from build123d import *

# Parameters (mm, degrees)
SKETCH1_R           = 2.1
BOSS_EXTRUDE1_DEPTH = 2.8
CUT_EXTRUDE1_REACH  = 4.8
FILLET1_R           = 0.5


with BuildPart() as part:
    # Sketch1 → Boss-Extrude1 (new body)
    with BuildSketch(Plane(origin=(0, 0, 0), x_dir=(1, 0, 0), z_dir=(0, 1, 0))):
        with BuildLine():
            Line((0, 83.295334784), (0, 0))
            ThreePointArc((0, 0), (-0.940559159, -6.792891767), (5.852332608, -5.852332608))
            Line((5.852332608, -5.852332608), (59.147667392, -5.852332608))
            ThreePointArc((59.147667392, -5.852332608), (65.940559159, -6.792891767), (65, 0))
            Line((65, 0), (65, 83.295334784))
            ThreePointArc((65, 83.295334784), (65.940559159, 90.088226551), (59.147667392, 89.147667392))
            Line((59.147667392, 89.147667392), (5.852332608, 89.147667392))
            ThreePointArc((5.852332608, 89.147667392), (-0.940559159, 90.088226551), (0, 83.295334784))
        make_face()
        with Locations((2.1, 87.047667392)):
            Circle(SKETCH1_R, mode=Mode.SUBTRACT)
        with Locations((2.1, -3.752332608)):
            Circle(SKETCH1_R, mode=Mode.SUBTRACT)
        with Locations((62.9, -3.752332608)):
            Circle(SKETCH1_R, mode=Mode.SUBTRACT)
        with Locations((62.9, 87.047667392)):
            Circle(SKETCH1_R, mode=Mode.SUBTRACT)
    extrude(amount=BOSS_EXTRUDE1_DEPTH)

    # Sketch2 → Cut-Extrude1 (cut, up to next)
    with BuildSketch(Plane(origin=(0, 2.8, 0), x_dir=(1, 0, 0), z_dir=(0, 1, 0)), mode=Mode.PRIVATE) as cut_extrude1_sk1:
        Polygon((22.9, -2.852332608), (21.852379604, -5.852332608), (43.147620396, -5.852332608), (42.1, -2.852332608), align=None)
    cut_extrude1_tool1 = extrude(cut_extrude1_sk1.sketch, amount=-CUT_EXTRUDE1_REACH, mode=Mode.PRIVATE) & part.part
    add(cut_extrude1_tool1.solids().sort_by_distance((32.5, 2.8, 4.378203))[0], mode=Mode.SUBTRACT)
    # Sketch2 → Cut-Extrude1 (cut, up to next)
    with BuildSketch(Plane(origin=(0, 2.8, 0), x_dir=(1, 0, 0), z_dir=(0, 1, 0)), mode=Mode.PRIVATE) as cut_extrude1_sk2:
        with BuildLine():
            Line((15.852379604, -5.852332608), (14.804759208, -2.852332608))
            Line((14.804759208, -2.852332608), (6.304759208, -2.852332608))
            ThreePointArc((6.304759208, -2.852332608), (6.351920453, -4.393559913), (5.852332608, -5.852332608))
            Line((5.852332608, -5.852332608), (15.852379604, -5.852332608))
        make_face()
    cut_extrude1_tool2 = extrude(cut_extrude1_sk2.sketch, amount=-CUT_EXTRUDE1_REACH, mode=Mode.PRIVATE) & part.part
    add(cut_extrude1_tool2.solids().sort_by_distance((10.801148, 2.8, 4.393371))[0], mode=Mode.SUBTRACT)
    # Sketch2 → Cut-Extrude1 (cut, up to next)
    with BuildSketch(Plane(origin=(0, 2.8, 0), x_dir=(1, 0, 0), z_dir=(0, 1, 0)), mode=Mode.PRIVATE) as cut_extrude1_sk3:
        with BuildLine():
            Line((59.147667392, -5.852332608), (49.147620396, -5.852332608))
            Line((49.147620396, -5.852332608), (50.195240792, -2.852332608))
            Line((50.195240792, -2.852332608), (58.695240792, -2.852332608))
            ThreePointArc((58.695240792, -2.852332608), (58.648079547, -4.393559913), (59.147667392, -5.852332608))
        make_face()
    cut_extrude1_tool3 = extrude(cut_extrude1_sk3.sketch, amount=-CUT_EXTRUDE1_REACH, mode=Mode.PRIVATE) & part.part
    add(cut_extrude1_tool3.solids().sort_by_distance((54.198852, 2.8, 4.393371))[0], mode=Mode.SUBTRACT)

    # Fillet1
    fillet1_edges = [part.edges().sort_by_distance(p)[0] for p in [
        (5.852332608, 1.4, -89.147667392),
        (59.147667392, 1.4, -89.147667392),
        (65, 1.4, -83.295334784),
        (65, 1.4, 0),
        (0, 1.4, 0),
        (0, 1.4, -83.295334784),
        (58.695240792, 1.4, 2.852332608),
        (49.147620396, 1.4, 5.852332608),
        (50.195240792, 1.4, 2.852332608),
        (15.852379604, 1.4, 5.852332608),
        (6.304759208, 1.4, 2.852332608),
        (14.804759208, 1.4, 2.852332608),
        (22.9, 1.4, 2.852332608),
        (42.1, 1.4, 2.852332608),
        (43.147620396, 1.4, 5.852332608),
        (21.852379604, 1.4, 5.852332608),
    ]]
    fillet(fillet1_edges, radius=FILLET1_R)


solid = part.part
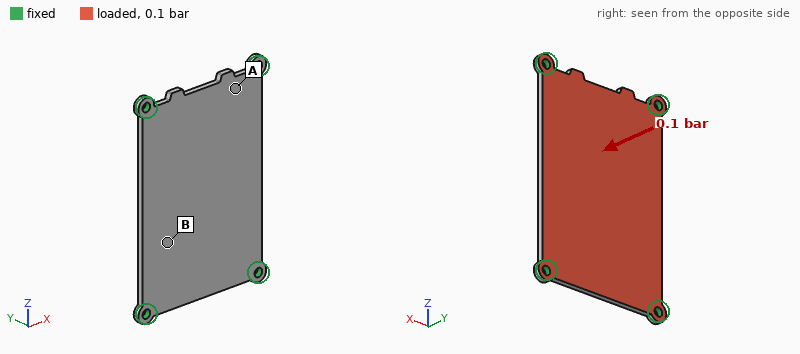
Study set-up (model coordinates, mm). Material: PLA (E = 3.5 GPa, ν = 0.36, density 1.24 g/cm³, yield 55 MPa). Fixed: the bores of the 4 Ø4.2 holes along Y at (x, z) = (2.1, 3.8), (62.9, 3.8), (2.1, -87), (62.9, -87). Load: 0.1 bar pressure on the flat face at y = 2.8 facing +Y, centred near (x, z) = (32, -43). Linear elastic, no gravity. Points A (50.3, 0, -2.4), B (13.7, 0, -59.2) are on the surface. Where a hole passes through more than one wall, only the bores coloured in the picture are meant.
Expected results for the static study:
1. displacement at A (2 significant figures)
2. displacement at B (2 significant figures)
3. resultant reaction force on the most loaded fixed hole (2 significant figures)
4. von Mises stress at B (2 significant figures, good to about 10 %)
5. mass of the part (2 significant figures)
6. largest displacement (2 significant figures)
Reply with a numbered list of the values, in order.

1. 0.097 mm
2. 0.36 mm
3. 16 N
4. 2.3 MPa
5. 21 g
6. 0.48 mm
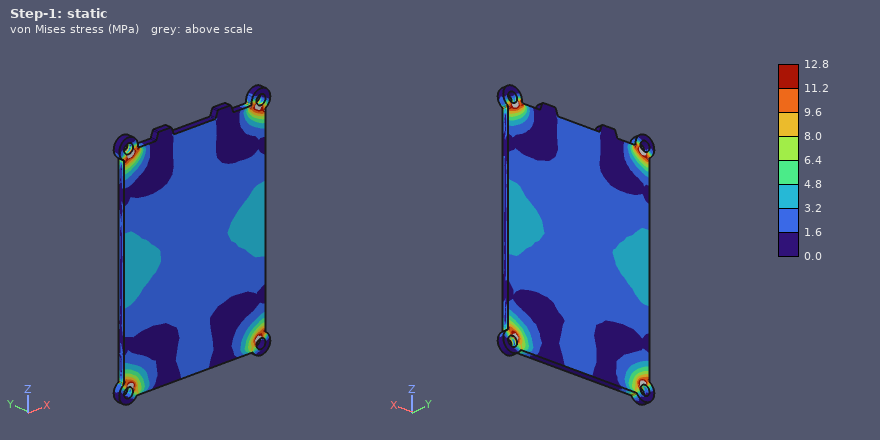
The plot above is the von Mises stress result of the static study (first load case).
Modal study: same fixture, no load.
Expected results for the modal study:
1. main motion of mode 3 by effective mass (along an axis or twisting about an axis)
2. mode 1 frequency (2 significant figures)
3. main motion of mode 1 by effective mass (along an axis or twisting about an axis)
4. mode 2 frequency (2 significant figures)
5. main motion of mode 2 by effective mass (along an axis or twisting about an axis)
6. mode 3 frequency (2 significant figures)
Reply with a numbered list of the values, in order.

1. twisting about X
2. 450 Hz
3. along Y
4. 780 Hz
5. twisting about Z
6. 1100 Hz
